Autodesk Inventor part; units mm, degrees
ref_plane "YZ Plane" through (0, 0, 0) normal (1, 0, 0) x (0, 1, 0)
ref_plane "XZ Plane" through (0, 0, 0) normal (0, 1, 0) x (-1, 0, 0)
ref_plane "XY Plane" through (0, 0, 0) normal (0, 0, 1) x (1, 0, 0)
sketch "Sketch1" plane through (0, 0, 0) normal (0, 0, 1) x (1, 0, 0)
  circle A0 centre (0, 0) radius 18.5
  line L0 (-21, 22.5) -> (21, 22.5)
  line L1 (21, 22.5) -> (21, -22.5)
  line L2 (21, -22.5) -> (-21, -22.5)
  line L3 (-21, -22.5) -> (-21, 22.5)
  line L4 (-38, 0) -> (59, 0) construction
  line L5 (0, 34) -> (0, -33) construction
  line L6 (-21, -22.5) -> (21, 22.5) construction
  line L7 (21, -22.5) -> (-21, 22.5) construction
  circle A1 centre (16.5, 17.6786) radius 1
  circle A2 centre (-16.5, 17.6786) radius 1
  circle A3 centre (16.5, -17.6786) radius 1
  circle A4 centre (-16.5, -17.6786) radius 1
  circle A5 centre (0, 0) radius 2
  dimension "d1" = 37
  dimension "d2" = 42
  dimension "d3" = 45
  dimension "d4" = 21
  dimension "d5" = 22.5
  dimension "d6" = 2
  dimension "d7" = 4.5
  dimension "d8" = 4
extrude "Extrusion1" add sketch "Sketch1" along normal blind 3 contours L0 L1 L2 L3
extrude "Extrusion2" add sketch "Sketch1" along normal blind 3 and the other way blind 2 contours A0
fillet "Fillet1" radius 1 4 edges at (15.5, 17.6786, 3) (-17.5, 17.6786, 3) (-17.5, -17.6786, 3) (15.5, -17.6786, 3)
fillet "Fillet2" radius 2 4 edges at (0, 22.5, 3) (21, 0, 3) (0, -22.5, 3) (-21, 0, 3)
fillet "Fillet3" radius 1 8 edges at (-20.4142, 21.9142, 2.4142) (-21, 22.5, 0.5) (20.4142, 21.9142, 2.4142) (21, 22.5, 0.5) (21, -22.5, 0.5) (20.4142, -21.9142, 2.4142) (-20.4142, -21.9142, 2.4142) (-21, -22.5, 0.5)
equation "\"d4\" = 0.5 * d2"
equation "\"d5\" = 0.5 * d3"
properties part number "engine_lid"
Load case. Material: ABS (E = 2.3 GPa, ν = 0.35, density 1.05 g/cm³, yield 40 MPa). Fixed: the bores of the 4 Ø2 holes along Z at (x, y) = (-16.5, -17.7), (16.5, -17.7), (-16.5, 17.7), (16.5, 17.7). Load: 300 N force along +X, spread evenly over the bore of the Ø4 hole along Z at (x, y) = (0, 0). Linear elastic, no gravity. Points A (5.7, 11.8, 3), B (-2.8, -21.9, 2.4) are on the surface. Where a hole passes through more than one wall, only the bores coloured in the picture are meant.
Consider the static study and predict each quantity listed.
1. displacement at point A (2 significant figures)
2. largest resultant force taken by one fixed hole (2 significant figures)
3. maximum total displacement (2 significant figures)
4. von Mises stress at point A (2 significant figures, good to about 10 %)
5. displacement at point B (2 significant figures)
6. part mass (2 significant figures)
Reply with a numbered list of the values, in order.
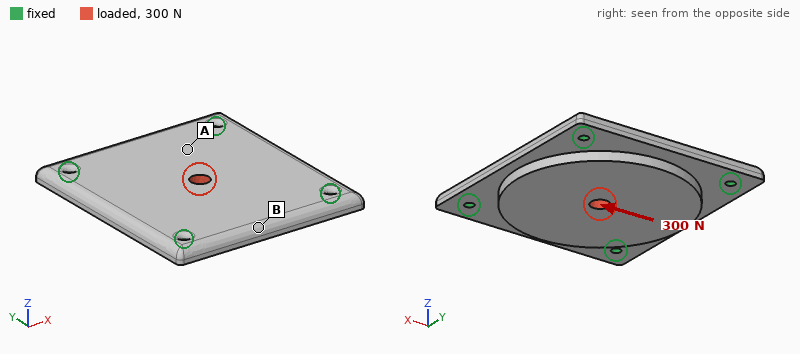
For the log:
1. 16 µm
2. 82 N
3. 36 µm
4. 1.7 MPa
5. 8.4 µm
6. 7.9 g
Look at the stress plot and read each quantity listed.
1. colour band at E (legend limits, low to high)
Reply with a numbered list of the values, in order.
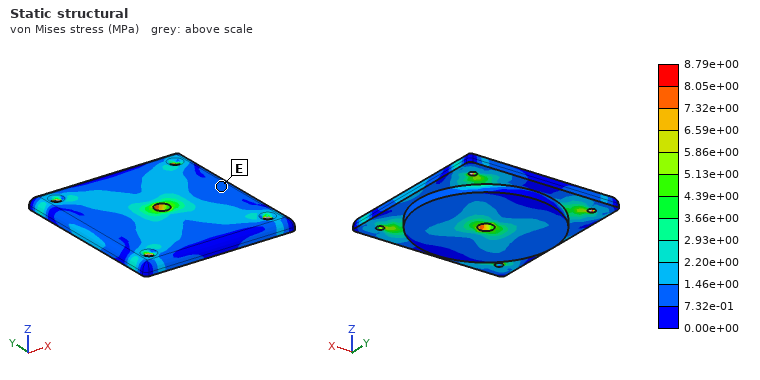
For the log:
1. 7.32e-01 to 1.46e+00 MPa
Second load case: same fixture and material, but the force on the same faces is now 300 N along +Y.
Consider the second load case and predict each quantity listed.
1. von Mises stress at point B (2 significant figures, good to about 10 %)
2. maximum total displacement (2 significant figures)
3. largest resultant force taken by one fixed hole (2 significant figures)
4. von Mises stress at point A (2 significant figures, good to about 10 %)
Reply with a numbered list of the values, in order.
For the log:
1. 1.5 MPa
2. 33 µm
3. 81 N
4. 1.5 MPa
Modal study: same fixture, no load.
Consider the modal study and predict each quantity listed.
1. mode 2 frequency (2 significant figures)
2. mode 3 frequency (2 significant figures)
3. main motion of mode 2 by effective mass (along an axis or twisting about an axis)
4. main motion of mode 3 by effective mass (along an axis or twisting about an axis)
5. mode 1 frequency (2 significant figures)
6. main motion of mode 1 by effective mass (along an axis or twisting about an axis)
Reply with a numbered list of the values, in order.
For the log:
1. 4000 Hz
2. 4300 Hz
3. twisting about Y
4. twisting about X
5. 2600 Hz
6. along Z
